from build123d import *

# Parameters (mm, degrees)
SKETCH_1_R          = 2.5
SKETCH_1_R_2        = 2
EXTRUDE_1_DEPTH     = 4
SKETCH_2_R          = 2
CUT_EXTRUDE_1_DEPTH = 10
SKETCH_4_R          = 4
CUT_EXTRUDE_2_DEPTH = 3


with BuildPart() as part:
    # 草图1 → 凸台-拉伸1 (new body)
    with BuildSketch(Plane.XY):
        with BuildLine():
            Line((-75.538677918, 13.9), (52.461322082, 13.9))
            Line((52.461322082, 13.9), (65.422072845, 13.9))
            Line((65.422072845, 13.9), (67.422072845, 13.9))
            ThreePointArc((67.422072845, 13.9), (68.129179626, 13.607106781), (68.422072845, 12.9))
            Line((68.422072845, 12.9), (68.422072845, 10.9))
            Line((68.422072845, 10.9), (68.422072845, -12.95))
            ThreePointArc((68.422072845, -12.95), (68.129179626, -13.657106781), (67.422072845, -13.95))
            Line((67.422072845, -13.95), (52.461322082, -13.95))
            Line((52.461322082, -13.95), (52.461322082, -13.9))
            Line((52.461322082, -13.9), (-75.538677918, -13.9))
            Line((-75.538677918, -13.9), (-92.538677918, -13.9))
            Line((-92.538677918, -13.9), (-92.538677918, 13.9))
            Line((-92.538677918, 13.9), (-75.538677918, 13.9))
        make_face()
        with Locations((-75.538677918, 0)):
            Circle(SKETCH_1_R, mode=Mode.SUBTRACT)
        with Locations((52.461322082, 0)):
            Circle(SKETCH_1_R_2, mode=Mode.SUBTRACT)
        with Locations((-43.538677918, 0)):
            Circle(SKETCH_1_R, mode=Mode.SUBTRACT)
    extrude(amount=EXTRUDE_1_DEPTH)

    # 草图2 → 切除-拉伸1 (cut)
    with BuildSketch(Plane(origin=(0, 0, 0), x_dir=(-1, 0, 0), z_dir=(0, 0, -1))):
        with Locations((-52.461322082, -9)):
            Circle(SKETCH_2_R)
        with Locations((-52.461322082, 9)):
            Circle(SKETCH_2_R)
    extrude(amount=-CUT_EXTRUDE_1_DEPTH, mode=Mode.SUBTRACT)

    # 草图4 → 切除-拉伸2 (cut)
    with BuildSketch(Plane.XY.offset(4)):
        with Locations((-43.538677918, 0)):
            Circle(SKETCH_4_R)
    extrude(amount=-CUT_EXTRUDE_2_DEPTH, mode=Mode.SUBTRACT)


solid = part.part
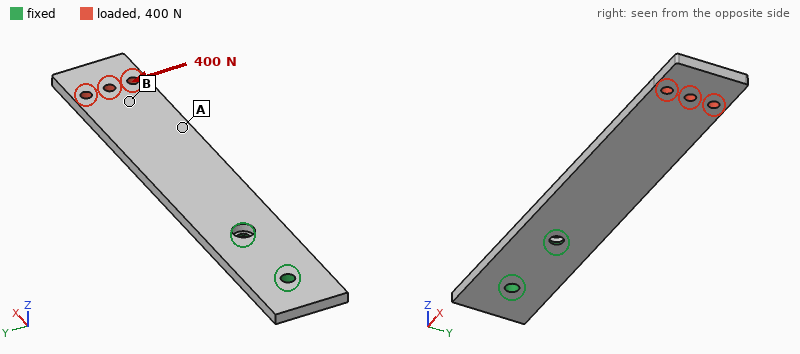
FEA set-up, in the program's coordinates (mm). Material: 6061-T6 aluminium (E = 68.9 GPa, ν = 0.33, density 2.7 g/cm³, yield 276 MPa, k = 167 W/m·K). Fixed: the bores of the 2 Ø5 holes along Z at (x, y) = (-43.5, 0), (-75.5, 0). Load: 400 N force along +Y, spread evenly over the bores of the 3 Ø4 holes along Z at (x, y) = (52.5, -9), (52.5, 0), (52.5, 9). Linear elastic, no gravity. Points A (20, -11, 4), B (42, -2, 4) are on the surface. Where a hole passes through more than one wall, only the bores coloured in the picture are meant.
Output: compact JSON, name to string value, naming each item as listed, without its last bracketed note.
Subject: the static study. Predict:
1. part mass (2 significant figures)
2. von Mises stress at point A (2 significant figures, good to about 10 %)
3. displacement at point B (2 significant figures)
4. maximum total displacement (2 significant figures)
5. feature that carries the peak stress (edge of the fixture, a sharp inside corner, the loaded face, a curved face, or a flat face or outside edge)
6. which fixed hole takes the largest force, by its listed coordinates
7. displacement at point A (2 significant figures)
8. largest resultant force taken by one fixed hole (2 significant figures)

{"part mass": "47 g", "von Mises stress at point A": "20 MPa", "displacement at point B": "0.35 mm", "maximum total displacement": "0.50 mm", "feature that carries the peak stress": "edge of the fixture", "which fixed hole takes the largest force, by its listed coordinates": "(-43.5, 0)", "displacement at point A": "0.24 mm", "largest resultant force taken by one fixed hole": "1.4 kN"}
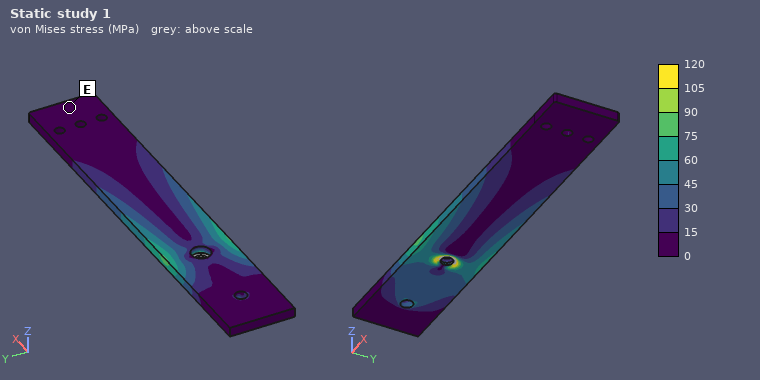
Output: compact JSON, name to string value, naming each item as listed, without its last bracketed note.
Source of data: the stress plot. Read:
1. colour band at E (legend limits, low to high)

{"colour band at E": "0 to 15 MPa"}
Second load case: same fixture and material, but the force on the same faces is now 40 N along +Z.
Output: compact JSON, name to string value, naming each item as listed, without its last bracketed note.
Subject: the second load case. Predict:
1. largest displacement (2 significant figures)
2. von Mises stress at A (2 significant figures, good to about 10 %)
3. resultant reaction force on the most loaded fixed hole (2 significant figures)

{"largest displacement": "1.7 mm", "von Mises stress at A": "18 MPa", "resultant reaction force on the most loaded fixed hole": "460 N"}
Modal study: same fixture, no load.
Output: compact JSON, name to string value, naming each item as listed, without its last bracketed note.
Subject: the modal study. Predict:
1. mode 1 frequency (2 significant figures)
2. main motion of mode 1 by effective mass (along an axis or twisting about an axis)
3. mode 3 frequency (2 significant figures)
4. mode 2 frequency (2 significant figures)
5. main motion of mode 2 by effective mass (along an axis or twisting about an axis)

{"mode 1 frequency": "240 Hz", "main motion of mode 1 by effective mass": "along Z", "mode 3 frequency": "1500 Hz", "mode 2 frequency": "1300 Hz", "main motion of mode 2 by effective mass": "along Y"}
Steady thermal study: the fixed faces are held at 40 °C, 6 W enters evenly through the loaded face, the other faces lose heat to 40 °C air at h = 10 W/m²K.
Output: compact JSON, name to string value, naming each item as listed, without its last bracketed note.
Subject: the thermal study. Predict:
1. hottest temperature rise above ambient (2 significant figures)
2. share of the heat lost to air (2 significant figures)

{"hottest temperature rise above ambient": "29 K", "share of the heat lost to air": "21 %"}
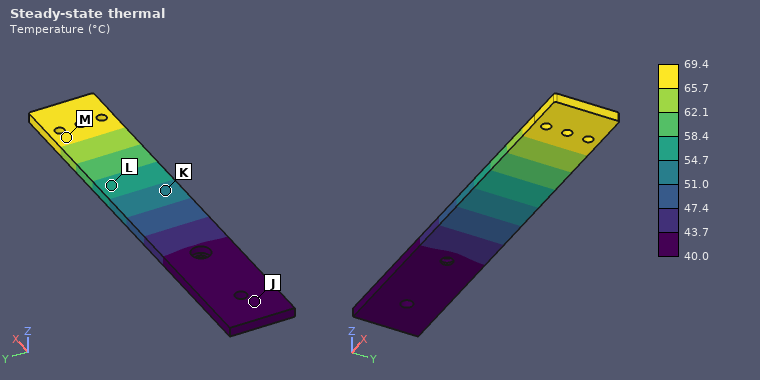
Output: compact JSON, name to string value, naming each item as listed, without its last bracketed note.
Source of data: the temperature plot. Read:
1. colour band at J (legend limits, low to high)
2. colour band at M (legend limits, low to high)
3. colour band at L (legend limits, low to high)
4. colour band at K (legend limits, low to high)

{"colour band at J": "40.0 to 43.7 °C", "colour band at M": "65.7 to 69.4 °C", "colour band at L": "54.7 to 58.4 °C", "colour band at K": "51.0 to 54.7 °C"}
